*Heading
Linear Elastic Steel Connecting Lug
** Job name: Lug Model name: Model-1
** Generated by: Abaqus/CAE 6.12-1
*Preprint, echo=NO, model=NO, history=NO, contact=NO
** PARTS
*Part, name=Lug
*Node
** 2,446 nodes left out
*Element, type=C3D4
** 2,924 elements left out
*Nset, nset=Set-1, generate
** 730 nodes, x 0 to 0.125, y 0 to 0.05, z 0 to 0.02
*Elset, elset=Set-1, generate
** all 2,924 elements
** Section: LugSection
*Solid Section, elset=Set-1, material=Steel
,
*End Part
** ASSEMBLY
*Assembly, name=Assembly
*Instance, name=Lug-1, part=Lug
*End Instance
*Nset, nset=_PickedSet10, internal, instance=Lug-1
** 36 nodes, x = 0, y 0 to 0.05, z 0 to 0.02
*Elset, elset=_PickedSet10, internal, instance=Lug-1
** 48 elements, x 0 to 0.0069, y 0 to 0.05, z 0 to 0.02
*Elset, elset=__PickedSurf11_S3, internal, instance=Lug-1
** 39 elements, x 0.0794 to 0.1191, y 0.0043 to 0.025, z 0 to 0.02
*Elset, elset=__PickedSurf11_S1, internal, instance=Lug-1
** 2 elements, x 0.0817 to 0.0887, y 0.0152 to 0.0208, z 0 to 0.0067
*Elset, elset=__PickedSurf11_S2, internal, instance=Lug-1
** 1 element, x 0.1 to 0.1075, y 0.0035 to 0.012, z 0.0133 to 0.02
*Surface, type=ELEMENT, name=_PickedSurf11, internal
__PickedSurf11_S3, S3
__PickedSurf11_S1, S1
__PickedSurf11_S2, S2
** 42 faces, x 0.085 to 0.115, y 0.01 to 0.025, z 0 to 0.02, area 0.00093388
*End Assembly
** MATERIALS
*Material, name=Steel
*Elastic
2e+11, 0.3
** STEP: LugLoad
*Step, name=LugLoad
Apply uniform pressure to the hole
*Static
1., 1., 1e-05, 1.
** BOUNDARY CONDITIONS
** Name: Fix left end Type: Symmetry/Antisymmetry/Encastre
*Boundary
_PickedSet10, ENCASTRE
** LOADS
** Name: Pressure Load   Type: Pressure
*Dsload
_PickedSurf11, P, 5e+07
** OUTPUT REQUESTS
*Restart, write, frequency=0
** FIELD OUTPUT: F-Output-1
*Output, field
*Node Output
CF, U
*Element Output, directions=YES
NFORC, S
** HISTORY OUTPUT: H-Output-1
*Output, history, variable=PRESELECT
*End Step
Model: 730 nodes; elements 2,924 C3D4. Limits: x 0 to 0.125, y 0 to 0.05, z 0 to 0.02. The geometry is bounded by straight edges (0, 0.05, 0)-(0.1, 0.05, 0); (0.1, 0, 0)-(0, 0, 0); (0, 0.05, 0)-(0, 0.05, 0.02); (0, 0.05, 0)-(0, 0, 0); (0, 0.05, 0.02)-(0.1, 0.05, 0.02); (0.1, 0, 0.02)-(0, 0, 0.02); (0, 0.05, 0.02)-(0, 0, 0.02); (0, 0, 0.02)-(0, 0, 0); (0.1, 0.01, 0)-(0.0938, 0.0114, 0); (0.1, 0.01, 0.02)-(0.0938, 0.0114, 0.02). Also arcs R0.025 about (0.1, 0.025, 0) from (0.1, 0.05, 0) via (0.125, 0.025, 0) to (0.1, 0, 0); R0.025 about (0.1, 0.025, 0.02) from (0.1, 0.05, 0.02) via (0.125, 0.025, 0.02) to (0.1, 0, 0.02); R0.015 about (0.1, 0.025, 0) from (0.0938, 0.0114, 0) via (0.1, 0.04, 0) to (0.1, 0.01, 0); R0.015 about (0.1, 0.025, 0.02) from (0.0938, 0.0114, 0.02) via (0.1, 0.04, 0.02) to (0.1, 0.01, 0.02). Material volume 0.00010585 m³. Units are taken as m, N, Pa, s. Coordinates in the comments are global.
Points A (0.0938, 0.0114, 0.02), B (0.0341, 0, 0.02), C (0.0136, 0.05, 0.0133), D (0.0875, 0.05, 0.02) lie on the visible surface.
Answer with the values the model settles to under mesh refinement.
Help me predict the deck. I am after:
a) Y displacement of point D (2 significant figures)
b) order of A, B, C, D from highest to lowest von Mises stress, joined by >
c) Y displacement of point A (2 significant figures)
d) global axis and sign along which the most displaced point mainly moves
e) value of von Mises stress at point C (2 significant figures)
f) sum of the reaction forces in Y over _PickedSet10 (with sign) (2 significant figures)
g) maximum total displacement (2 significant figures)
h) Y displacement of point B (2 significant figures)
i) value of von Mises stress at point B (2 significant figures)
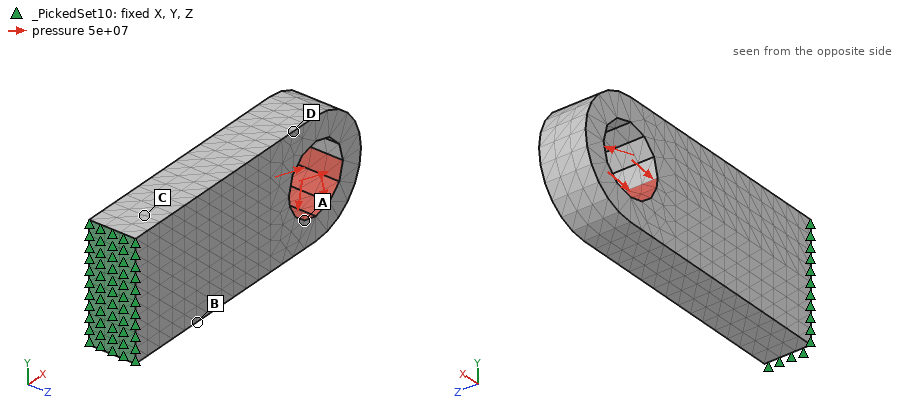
-2.3e-04 m
C > A > B > D
-2.7e-04 m
-Y
3.1e+08 Pa
30000 N
4.2e-04 m
-5.4e-05 m
2.4e+08 Pa
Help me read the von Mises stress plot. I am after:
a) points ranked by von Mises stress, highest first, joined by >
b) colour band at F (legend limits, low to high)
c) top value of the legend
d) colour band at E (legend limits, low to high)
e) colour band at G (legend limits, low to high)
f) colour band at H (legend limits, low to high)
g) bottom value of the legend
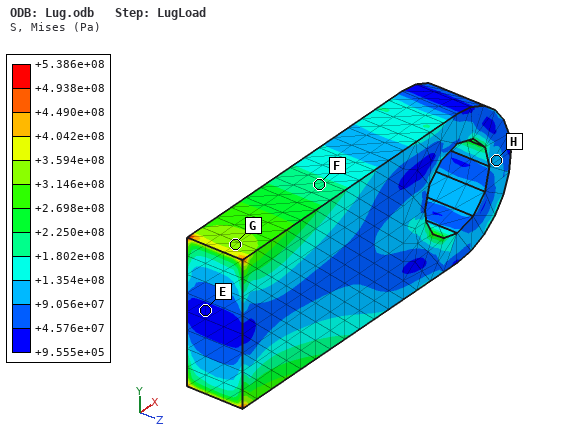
G > F > H > E
+1.802e+08 to +2.250e+08 Pa
+5.386e+08 Pa
+9.555e+05 to +4.576e+07 Pa
+3.146e+08 to +3.594e+08 Pa
+9.056e+07 to +1.354e+08 Pa
+9.555e+05 Pa
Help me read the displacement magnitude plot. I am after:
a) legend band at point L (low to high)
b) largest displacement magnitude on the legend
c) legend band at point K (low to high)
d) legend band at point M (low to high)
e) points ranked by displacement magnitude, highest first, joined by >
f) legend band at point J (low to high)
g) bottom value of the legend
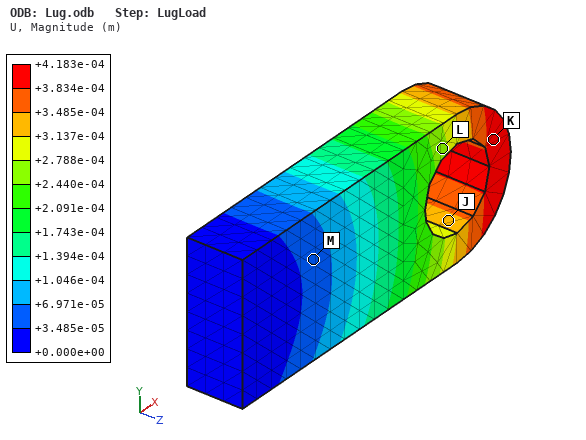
+2.440e-04 to +2.788e-04 m
+4.183e-04 m
+3.834e-04 to +4.183e-04 m
+3.485e-05 to +6.971e-05 m
K > J > L > M
+3.137e-04 to +3.485e-04 m
+0.000e+00 m
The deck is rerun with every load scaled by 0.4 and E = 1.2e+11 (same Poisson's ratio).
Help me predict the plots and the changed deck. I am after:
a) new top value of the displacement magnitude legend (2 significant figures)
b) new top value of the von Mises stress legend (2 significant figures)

2.8e-04 m
2.2e+08 Pa
